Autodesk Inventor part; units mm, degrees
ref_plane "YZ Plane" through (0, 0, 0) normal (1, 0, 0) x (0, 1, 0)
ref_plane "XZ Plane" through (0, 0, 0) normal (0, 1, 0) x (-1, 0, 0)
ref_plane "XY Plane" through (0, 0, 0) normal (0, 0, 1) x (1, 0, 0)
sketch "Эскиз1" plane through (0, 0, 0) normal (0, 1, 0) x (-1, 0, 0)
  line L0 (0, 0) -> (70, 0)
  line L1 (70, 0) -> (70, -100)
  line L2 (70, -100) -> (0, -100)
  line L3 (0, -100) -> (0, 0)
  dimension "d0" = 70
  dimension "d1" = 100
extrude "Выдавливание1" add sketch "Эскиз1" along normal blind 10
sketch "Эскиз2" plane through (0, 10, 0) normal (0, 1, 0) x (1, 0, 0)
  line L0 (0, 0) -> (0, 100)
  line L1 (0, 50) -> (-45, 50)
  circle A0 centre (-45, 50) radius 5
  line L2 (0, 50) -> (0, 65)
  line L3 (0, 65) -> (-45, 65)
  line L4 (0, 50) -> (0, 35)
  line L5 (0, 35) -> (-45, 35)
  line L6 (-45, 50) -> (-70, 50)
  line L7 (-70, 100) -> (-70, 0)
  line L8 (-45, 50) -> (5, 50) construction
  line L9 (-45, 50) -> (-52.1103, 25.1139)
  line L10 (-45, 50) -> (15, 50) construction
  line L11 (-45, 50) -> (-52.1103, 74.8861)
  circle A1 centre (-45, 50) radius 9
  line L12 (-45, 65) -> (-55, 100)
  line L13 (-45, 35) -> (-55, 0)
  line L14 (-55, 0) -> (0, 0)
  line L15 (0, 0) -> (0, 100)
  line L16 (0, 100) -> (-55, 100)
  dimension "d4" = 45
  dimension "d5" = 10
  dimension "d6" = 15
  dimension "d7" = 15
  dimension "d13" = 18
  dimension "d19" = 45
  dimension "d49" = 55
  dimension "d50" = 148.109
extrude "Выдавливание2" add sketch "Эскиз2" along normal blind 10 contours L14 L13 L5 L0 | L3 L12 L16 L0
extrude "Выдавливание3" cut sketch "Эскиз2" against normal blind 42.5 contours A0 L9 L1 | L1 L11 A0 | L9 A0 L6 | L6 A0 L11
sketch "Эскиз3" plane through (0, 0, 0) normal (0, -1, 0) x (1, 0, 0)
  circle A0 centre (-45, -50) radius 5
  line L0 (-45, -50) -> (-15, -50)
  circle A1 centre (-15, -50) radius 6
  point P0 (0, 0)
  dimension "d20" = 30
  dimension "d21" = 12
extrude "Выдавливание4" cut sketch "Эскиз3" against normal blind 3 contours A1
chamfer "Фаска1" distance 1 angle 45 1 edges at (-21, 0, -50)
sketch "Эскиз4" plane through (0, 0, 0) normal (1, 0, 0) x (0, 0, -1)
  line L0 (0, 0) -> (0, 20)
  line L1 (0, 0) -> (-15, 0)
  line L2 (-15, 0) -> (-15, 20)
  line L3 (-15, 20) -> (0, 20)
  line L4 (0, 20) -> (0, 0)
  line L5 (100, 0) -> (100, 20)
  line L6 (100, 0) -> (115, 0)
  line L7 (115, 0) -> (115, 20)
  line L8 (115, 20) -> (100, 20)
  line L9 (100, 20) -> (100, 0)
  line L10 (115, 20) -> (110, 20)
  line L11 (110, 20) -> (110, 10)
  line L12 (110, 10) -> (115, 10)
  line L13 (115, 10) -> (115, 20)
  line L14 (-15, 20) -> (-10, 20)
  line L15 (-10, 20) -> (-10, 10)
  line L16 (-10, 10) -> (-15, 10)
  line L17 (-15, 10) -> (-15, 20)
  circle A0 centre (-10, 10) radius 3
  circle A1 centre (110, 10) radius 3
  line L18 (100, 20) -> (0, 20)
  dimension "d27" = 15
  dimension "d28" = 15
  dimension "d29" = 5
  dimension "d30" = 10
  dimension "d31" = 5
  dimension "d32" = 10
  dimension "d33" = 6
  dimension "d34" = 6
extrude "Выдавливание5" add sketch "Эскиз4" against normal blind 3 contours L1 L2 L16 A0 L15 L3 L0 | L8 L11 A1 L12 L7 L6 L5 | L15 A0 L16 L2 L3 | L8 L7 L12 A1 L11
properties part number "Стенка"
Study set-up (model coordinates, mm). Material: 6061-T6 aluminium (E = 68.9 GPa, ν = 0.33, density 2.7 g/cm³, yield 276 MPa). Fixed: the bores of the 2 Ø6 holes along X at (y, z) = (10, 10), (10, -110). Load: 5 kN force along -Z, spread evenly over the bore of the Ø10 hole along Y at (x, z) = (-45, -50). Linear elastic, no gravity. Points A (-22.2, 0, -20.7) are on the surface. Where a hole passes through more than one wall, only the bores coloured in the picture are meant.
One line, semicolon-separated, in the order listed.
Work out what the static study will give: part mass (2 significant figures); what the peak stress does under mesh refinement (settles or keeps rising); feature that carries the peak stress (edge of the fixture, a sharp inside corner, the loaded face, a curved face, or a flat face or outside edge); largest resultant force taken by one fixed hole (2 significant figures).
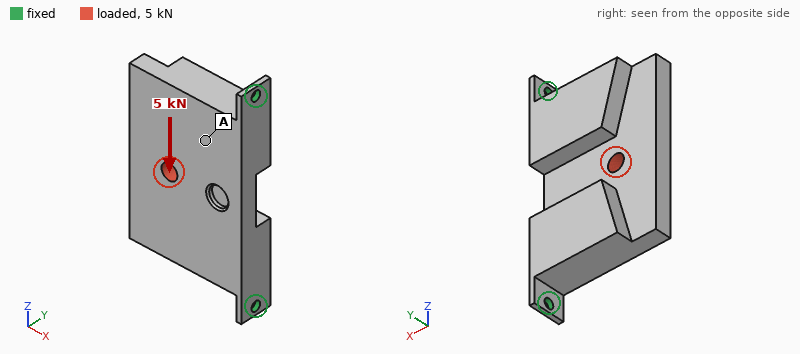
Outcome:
280 g; keeps rising; edge of the fixture; 3.2 kN
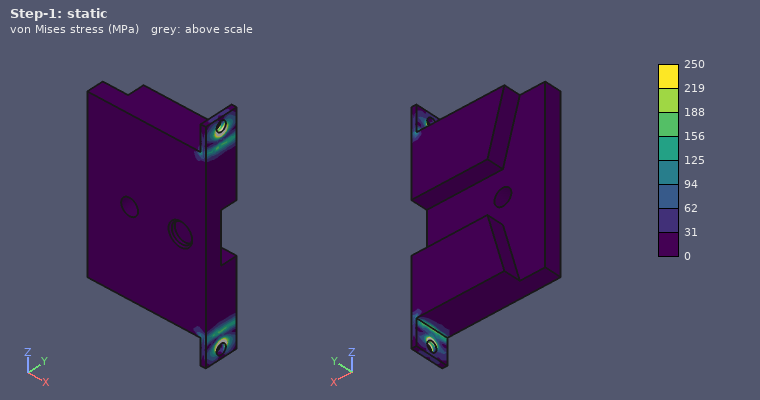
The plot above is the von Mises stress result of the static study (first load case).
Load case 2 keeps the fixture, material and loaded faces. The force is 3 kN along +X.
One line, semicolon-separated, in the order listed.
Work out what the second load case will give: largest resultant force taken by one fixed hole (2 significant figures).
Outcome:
1.8 kN
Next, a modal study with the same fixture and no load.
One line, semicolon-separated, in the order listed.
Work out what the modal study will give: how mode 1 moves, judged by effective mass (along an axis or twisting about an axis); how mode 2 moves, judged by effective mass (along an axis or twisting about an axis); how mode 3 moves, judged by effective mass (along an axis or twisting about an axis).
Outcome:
along Y; along X; along Z
